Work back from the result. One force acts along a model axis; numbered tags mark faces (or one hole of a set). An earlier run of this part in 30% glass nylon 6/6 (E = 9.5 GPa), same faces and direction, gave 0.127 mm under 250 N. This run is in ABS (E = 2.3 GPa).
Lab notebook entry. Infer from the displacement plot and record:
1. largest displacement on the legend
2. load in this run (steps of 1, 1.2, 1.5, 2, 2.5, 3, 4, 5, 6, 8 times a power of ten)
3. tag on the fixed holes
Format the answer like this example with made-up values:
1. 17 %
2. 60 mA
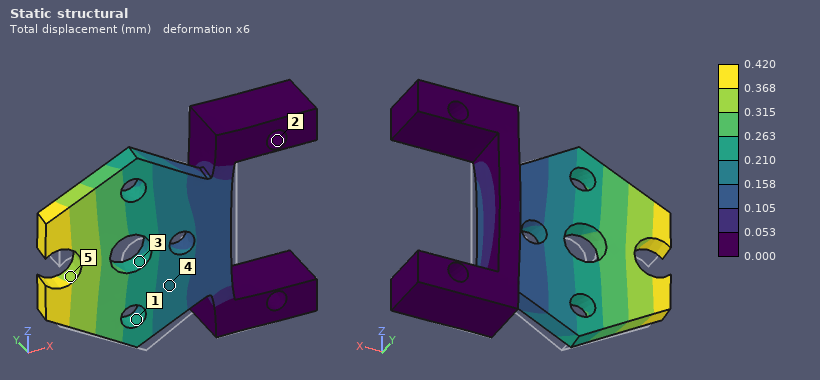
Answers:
1. 0.420 mm
2. 200 N
3. 2
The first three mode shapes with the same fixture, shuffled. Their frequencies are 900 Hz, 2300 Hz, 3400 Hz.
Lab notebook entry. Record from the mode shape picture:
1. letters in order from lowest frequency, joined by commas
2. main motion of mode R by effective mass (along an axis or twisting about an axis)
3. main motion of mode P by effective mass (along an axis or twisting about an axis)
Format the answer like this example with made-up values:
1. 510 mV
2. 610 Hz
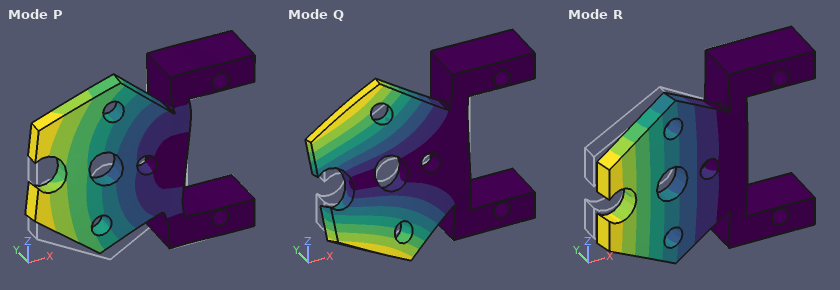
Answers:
1. R, Q, P
2. along Y
3. along Z
